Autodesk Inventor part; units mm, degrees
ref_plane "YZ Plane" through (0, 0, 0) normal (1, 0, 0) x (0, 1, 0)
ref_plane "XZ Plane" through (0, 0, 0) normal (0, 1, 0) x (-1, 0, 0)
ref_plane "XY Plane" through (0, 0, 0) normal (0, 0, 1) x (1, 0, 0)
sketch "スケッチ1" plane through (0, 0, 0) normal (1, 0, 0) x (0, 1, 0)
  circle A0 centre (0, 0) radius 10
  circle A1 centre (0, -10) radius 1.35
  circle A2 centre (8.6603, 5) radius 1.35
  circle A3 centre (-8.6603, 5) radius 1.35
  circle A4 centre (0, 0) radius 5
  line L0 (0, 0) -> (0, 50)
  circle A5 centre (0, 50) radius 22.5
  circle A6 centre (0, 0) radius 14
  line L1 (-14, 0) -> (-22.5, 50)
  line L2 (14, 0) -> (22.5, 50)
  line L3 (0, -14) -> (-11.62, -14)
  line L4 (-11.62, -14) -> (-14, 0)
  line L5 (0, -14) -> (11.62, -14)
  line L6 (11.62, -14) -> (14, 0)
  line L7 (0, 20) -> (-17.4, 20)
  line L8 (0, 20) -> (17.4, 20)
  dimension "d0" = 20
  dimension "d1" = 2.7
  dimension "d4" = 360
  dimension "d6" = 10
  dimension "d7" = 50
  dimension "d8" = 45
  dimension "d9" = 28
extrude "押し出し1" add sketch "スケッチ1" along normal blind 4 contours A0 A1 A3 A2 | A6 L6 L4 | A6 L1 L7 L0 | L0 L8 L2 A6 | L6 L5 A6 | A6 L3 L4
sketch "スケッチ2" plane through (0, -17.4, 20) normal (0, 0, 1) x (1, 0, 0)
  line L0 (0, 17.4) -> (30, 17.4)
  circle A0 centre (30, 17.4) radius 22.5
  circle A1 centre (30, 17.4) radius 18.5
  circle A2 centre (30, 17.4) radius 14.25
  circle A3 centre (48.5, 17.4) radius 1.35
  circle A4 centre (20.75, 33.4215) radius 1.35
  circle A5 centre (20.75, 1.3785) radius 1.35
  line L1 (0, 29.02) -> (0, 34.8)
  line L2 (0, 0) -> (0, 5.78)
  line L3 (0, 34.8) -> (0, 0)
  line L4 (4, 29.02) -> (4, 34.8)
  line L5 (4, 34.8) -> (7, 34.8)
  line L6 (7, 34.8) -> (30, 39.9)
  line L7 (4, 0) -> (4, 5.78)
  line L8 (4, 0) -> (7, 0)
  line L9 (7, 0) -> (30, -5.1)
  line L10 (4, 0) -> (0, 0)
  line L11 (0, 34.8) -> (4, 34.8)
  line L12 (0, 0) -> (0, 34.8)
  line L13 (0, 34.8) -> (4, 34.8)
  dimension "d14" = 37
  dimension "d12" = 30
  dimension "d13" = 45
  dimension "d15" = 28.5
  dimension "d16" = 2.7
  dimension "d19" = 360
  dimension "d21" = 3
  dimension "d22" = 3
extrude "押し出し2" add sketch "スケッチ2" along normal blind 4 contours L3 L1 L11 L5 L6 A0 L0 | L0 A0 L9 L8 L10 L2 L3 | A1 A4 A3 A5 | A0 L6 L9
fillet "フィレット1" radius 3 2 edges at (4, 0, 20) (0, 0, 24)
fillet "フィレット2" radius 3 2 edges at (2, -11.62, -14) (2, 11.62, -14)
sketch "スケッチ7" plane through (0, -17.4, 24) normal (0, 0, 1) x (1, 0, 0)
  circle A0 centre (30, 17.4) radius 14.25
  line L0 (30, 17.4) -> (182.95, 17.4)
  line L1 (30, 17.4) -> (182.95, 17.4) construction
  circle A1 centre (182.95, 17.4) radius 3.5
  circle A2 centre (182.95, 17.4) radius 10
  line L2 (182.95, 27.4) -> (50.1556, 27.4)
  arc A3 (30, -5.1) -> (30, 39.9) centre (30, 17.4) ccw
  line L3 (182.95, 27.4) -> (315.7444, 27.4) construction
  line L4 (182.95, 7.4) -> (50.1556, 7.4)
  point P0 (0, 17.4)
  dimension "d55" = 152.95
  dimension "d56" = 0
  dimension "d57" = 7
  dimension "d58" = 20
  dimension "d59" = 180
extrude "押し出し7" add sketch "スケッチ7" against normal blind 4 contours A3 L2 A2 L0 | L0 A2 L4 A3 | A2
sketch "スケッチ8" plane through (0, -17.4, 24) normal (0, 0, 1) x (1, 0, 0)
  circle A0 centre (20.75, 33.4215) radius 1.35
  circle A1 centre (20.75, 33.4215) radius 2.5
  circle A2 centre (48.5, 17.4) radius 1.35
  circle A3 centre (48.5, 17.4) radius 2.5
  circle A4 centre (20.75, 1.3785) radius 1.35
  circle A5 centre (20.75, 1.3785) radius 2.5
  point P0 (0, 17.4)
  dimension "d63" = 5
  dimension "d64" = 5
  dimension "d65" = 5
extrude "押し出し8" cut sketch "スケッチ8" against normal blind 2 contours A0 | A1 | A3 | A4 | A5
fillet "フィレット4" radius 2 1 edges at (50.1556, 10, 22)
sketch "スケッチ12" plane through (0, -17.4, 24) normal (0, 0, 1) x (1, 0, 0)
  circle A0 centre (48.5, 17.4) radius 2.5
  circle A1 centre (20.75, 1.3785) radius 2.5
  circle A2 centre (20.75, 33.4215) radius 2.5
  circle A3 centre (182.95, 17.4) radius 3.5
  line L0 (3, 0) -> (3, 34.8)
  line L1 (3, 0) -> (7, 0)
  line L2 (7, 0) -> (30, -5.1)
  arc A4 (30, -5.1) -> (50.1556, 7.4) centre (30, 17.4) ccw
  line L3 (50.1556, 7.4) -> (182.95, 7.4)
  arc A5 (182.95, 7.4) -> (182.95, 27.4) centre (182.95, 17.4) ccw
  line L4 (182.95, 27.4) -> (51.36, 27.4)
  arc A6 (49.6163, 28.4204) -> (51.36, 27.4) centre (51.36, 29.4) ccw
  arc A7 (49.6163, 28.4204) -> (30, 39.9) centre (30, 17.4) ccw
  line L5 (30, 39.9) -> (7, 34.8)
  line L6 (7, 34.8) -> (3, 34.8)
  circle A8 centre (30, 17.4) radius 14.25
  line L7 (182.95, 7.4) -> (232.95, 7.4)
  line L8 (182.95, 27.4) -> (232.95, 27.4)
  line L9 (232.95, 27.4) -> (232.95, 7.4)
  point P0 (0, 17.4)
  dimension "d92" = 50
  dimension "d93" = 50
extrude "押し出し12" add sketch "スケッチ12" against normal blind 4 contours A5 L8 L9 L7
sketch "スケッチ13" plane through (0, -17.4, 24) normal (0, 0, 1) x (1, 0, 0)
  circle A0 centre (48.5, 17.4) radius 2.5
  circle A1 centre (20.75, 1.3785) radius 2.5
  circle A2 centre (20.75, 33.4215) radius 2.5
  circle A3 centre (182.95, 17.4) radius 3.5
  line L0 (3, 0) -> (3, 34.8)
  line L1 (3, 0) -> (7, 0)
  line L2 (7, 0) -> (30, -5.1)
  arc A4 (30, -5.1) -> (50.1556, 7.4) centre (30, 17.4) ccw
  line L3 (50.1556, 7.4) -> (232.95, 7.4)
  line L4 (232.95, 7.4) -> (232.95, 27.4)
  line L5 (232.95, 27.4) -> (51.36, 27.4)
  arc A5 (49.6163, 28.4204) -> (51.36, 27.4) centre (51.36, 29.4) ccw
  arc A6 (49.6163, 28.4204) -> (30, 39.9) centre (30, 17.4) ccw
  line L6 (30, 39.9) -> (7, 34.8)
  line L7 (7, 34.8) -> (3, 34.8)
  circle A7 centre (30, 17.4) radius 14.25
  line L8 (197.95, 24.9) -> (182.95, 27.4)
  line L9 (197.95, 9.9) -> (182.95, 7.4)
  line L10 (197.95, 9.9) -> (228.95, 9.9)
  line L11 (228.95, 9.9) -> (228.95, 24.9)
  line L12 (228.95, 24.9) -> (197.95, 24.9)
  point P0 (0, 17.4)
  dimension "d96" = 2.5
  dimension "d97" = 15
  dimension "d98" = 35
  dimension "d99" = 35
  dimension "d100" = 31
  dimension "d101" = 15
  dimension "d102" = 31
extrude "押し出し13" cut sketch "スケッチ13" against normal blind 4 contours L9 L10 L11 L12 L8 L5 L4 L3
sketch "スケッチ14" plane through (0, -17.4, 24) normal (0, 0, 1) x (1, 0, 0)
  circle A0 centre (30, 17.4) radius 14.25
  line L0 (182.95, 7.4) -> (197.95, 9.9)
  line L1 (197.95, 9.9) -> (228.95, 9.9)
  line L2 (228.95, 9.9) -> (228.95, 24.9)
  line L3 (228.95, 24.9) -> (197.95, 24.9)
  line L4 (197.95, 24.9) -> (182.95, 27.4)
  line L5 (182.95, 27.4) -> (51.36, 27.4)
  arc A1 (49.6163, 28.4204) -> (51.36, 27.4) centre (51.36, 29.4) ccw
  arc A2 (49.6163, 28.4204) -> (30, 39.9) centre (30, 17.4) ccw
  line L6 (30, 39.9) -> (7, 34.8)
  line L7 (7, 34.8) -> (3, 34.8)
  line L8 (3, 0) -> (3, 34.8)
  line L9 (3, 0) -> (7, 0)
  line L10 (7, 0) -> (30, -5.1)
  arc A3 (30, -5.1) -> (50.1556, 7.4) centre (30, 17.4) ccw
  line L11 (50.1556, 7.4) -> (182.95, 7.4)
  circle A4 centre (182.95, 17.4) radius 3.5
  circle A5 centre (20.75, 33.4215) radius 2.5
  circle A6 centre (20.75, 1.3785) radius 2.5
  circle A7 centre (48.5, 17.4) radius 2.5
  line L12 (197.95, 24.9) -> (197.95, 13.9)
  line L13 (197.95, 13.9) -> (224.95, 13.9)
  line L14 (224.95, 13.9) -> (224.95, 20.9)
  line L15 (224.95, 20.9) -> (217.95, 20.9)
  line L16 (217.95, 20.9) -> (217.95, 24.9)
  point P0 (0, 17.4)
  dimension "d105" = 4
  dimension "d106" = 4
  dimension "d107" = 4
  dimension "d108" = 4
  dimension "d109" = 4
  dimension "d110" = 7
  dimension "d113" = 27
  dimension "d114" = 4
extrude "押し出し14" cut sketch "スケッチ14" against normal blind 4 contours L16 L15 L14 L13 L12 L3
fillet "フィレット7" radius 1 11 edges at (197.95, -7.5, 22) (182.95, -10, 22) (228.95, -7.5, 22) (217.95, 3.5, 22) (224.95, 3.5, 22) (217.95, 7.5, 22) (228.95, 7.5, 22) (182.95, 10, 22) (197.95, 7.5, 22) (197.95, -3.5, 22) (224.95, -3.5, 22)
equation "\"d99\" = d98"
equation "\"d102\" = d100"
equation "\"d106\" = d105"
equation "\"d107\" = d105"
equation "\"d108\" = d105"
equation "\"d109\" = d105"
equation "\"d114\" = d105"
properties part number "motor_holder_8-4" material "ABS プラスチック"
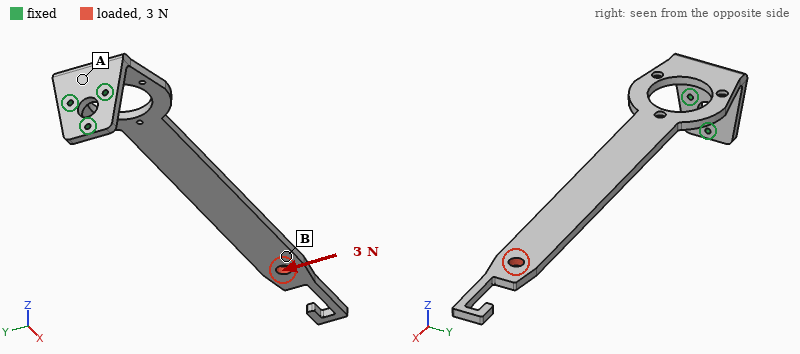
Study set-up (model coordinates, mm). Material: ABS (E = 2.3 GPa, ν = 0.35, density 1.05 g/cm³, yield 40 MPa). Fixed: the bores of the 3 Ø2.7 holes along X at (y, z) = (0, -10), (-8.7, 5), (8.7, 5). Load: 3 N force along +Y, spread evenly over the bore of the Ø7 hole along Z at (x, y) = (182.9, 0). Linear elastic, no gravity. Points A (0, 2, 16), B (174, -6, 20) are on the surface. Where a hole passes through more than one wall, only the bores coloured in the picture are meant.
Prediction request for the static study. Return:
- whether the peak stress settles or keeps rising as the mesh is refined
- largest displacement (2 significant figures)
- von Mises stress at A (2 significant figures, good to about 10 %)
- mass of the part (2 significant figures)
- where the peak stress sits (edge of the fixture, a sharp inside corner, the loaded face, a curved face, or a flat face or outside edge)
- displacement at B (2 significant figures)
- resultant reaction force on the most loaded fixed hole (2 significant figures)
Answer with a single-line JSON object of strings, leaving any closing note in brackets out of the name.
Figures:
{"whether the peak stress settles or keeps rising as the mesh is refined": "keeps rising", "largest displacement": "2.5 mm", "von Mises stress at A": "2.9 MPa", "mass of the part": "22 g", "where the peak stress sits": "edge of the fixture", "displacement at B": "1.8 mm", "resultant reaction force on the most loaded fixed hole": "26 N"}
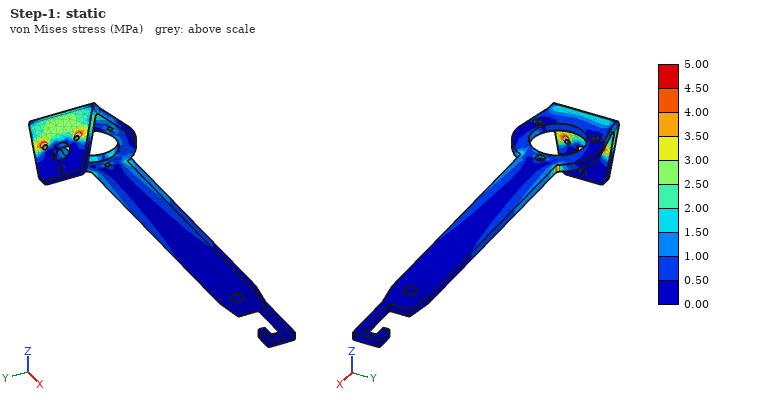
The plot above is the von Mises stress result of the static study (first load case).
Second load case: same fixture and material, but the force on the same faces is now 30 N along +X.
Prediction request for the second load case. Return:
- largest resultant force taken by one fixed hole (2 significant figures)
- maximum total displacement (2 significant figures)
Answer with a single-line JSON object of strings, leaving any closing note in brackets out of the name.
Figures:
{"largest resultant force taken by one fixed hole": "17 N", "maximum total displacement": "2.8 mm"}
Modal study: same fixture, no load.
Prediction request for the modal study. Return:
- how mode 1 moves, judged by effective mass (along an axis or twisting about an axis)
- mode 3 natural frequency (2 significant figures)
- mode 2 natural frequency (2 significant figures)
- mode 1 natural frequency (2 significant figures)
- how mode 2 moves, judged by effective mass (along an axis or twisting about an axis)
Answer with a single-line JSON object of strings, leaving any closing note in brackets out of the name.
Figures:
{"how mode 1 moves, judged by effective mass": "along Z", "mode 3 natural frequency": "120 Hz", "mode 2 natural frequency": "77 Hz", "mode 1 natural frequency": "20 Hz", "how mode 2 moves, judged by effective mass": "along Y"}
